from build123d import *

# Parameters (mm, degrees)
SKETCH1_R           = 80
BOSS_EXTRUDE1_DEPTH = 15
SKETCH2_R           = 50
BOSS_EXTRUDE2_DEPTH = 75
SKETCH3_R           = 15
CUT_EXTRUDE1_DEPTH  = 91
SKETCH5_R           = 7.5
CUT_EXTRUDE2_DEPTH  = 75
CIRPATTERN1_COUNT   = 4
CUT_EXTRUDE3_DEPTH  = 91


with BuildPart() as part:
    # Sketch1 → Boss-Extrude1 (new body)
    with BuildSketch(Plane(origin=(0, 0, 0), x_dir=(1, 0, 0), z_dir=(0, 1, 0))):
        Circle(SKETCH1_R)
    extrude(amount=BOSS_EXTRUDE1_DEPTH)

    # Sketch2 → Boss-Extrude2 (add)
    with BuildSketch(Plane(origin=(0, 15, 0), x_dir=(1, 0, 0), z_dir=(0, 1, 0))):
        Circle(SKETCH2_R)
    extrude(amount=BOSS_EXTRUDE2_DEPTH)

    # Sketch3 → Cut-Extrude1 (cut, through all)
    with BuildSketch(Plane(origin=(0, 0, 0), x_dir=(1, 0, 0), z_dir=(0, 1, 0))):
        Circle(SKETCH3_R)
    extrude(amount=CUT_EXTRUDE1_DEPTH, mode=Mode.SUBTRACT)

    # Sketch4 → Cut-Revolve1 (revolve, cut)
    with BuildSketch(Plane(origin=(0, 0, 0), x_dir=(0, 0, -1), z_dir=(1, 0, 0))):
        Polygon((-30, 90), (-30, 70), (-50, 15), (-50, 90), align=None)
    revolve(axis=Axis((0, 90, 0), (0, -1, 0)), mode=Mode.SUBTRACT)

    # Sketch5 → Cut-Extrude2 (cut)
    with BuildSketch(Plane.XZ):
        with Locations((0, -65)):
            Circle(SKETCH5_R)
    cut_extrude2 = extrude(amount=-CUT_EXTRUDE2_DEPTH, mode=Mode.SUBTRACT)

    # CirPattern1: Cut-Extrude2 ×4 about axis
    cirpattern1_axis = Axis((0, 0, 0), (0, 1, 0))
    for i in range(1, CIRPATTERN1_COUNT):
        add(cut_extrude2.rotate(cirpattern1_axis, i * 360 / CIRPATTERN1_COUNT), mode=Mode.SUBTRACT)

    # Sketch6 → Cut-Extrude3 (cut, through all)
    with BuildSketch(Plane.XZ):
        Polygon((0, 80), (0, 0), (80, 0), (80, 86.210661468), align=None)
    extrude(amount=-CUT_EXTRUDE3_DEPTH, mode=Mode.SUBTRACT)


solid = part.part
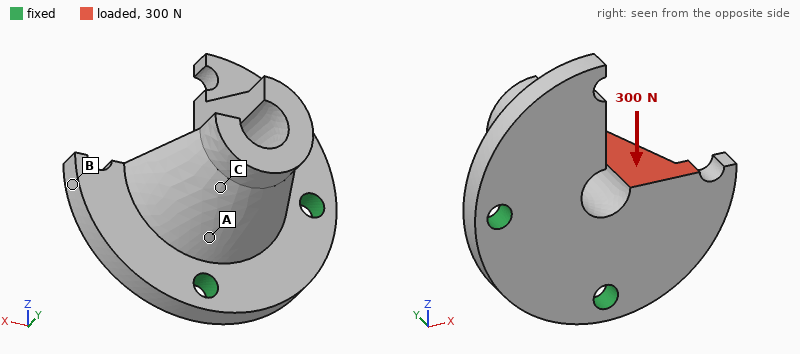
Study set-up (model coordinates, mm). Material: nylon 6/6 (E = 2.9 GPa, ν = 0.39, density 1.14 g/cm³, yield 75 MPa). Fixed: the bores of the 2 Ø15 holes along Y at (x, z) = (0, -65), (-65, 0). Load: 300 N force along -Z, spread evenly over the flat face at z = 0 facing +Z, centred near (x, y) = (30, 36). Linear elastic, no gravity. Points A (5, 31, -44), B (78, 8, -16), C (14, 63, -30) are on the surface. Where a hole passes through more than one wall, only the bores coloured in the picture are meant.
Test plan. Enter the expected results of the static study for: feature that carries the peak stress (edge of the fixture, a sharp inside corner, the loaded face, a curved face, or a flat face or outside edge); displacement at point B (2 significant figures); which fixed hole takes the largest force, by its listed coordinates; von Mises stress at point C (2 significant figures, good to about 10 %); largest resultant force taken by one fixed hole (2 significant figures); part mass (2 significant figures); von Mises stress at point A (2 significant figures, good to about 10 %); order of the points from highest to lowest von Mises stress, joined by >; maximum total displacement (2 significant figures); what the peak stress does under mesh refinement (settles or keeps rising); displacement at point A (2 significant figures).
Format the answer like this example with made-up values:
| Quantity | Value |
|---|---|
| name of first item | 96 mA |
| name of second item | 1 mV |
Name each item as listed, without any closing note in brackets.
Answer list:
| Quantity | Value |
|---|---|
| feature that carries the peak stress | edge of the fixture |
| displacement at point B | 0.080 mm |
| which fixed hole takes the largest force, by its listed coordinates | (0, -65) |
| von Mises stress at point C | 0.43 MPa |
| largest resultant force taken by one fixed hole | 320 N |
| part mass | 480 g |
| von Mises stress at point A | 0.55 MPa |
| order of the points from highest to lowest von Mises stress, joined by > | A > C > B |
| maximum total displacement | 0.13 mm |
| what the peak stress does under mesh refinement | keeps rising |
| displacement at point A | 0.030 mm |
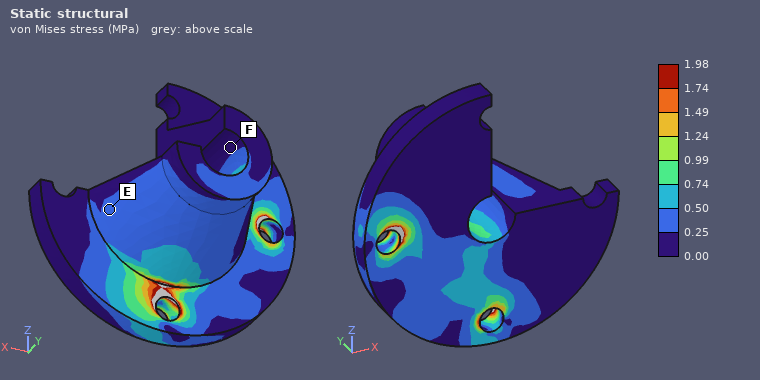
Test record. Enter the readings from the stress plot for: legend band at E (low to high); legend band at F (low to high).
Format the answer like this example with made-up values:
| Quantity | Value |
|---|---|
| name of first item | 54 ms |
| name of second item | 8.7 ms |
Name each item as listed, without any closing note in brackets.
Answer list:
| Quantity | Value |
|---|---|
| legend band at E | 0.25 to 0.50 MPa |
| legend band at F | 0.00 to 0.25 MPa |
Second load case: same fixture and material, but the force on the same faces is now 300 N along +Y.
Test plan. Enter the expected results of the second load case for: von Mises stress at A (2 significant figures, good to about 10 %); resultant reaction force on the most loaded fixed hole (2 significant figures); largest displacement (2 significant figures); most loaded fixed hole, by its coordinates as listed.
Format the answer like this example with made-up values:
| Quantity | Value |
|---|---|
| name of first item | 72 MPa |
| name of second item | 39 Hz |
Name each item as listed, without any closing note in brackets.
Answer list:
| Quantity | Value |
|---|---|
| von Mises stress at A | 0.99 MPa |
| resultant reaction force on the most loaded fixed hole | 230 N |
| largest displacement | 0.33 mm |
| most loaded fixed hole, by its coordinates as listed | (0, -65) |
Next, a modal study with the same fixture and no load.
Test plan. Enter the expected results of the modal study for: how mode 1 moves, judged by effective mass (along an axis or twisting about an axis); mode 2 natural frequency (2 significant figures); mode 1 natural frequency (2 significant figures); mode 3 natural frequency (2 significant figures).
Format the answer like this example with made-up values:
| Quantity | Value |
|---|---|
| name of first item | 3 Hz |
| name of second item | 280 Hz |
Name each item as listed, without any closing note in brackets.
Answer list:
| Quantity | Value |
|---|---|
| how mode 1 moves, judged by effective mass | along Y |
| mode 2 natural frequency | 1000 Hz |
| mode 1 natural frequency | 390 Hz |
| mode 3 natural frequency | 1300 Hz |
